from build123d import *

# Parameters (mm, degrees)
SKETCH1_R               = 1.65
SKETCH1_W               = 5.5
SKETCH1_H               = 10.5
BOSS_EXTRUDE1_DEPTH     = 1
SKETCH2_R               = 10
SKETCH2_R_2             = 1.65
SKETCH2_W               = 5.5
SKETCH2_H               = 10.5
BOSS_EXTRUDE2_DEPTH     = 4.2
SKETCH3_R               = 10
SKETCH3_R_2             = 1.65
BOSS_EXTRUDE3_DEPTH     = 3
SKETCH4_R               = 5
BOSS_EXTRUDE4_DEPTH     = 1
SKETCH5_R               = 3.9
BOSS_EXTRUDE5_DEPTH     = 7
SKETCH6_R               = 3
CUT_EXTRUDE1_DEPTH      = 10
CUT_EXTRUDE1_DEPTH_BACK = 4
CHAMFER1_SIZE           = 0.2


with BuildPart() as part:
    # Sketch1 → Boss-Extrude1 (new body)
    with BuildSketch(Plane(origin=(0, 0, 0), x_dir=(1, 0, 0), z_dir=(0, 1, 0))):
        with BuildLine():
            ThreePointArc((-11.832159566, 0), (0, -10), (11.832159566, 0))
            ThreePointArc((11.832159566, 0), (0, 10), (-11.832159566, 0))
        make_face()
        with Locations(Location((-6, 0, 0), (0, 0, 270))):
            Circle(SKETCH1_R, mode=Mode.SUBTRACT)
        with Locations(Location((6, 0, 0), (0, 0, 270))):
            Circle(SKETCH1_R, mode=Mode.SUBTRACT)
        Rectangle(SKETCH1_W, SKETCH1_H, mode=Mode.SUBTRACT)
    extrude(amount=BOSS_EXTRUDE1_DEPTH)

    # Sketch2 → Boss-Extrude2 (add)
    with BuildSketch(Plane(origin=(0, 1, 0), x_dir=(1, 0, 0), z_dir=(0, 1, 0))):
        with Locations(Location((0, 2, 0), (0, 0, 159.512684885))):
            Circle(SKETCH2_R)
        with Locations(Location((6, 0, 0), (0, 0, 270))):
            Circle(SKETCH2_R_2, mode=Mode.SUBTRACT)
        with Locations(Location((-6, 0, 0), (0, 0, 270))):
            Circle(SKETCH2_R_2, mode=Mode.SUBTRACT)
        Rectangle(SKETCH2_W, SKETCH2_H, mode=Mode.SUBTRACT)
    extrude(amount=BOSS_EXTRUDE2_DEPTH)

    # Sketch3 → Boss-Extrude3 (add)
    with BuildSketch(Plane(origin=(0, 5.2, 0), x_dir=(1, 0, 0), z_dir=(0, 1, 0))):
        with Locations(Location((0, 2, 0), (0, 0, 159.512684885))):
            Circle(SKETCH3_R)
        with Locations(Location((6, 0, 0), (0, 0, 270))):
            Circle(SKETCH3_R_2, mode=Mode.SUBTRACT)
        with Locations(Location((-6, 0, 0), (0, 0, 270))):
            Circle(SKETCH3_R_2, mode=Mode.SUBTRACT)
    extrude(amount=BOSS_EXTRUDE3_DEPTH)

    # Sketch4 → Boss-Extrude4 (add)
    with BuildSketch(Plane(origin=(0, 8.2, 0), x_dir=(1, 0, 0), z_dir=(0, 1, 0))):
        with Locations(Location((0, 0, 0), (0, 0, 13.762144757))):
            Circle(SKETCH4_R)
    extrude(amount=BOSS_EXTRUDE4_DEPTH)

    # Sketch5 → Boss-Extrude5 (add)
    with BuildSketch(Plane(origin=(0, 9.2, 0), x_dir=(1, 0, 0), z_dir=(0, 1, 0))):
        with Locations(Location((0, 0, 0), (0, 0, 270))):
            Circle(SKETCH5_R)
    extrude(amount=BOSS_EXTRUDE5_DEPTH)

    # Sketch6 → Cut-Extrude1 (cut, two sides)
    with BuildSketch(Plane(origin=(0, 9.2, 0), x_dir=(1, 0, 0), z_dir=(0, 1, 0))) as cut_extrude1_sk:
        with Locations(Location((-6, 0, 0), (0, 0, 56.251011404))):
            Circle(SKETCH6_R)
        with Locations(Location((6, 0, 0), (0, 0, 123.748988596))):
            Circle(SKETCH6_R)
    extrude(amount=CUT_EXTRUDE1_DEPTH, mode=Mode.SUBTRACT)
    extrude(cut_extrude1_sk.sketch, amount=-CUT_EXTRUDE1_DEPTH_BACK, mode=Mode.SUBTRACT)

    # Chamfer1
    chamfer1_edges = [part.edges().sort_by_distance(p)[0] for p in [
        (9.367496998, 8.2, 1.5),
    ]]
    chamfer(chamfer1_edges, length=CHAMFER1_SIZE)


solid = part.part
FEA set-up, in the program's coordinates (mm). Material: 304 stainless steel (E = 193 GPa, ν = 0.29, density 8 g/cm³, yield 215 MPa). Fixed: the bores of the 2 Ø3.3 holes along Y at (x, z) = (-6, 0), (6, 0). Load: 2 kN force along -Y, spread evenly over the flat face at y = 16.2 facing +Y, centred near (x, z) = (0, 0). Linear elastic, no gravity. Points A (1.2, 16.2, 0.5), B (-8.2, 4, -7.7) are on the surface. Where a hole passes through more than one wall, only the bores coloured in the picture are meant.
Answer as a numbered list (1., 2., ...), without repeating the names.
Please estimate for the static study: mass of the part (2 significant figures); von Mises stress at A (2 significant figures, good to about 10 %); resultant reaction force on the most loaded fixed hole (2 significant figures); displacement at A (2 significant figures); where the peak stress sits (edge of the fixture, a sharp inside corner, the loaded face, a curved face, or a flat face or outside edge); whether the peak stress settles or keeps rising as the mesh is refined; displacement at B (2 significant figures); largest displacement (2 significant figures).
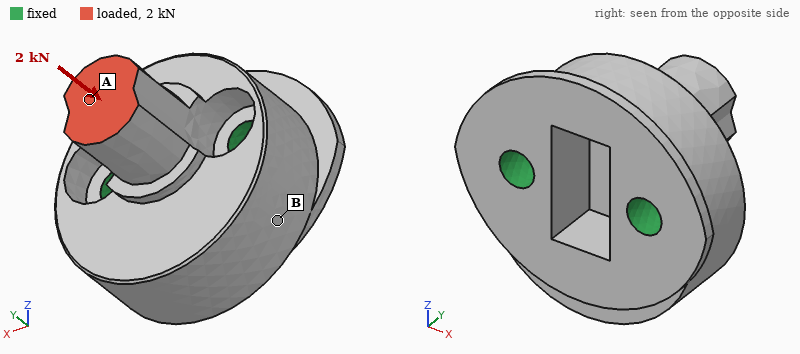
1. 19 g
2. 46 MPa
3. 1.0 kN
4. 3.9 µm
5. a sharp inside corner
6. keeps rising
7. 0.83 µm
8. 4.0 µm
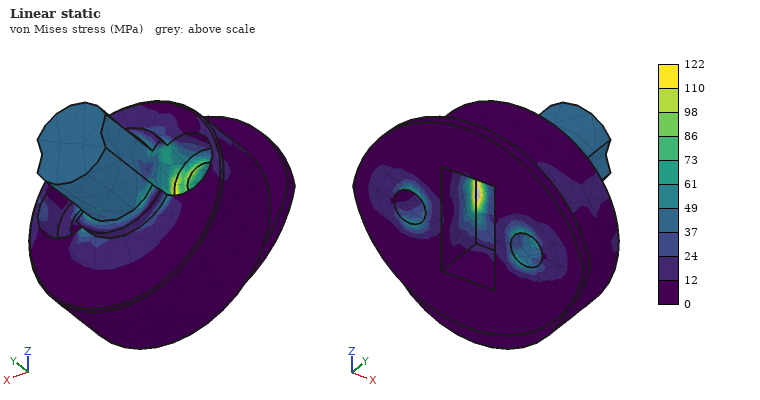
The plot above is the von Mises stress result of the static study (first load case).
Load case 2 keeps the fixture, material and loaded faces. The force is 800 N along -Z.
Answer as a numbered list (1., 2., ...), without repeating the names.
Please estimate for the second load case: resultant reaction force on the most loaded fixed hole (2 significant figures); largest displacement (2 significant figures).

1. 400 N
2. 15 µm
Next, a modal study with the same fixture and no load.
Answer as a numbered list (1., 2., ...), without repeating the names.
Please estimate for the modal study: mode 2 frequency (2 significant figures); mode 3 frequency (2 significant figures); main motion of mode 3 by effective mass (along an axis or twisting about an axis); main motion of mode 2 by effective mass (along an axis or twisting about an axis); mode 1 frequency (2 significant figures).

1. 37 kHz
2. 45 kHz
3. along Y
4. along X
5. 24 kHz
